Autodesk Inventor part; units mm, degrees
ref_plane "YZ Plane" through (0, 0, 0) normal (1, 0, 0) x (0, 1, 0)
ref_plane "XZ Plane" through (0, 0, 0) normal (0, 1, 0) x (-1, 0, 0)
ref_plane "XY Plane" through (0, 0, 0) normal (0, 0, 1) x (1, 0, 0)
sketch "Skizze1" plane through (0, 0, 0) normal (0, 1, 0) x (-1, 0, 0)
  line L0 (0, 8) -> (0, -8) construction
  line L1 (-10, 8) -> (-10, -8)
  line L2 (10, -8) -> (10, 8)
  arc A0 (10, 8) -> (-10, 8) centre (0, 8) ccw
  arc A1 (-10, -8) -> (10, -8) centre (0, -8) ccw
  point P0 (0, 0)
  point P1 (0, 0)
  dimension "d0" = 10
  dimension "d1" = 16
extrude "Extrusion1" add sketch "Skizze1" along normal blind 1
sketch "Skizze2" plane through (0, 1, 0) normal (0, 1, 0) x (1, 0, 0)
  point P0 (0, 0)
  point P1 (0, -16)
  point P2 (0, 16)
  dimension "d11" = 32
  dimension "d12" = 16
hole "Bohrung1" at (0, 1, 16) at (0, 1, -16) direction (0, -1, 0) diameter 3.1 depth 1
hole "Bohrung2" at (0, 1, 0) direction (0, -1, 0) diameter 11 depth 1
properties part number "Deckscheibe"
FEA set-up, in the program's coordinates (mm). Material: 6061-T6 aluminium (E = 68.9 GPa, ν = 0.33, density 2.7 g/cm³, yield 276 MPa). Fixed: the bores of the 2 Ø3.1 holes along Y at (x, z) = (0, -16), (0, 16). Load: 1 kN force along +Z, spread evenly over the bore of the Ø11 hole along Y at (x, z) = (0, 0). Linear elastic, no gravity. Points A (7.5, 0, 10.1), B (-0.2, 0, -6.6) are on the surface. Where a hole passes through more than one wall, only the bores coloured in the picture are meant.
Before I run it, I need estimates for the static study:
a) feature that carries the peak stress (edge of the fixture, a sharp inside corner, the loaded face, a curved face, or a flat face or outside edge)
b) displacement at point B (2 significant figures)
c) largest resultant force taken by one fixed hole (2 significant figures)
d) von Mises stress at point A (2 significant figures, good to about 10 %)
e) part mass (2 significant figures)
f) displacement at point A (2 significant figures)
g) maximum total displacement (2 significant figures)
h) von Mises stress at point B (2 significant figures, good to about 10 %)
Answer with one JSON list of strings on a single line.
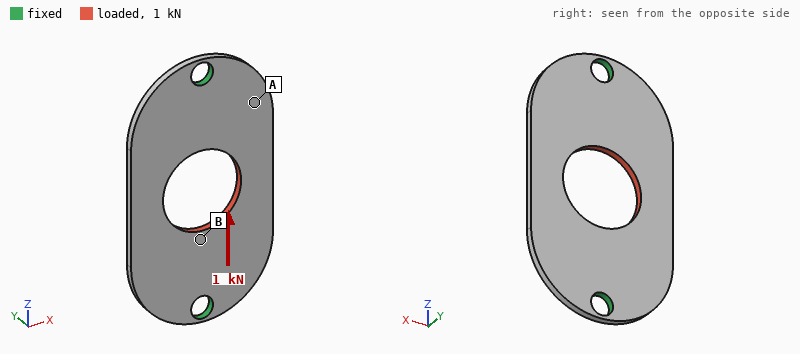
["edge of the fixture", "6.5 µm", "500 N", "13 MPa", "1.4 g", "7.1 µm", "11 µm", "41 MPa"]
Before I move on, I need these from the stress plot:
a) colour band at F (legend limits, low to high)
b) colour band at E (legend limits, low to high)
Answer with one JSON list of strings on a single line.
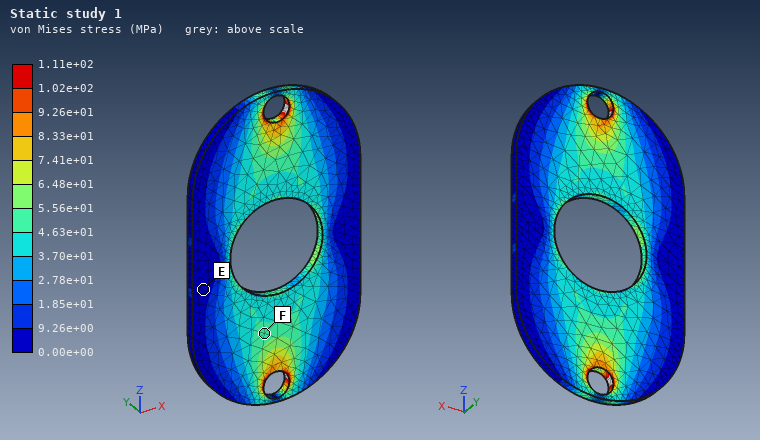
["4.63e+01 to 5.56e+01 MPa", "0.00e+00 to 9.26e+00 MPa"]
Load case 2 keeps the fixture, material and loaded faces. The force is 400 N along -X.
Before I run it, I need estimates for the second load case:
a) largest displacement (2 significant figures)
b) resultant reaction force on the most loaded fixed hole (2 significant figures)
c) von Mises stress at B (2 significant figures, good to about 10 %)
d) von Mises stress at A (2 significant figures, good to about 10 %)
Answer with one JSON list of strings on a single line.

["12 µm", "200 N", "24 MPa", "15 MPa"]
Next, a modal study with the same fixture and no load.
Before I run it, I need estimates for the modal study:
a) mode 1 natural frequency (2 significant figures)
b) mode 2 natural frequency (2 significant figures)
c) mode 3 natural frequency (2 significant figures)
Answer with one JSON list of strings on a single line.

["4600 Hz", "4800 Hz", "10 kHz"]
